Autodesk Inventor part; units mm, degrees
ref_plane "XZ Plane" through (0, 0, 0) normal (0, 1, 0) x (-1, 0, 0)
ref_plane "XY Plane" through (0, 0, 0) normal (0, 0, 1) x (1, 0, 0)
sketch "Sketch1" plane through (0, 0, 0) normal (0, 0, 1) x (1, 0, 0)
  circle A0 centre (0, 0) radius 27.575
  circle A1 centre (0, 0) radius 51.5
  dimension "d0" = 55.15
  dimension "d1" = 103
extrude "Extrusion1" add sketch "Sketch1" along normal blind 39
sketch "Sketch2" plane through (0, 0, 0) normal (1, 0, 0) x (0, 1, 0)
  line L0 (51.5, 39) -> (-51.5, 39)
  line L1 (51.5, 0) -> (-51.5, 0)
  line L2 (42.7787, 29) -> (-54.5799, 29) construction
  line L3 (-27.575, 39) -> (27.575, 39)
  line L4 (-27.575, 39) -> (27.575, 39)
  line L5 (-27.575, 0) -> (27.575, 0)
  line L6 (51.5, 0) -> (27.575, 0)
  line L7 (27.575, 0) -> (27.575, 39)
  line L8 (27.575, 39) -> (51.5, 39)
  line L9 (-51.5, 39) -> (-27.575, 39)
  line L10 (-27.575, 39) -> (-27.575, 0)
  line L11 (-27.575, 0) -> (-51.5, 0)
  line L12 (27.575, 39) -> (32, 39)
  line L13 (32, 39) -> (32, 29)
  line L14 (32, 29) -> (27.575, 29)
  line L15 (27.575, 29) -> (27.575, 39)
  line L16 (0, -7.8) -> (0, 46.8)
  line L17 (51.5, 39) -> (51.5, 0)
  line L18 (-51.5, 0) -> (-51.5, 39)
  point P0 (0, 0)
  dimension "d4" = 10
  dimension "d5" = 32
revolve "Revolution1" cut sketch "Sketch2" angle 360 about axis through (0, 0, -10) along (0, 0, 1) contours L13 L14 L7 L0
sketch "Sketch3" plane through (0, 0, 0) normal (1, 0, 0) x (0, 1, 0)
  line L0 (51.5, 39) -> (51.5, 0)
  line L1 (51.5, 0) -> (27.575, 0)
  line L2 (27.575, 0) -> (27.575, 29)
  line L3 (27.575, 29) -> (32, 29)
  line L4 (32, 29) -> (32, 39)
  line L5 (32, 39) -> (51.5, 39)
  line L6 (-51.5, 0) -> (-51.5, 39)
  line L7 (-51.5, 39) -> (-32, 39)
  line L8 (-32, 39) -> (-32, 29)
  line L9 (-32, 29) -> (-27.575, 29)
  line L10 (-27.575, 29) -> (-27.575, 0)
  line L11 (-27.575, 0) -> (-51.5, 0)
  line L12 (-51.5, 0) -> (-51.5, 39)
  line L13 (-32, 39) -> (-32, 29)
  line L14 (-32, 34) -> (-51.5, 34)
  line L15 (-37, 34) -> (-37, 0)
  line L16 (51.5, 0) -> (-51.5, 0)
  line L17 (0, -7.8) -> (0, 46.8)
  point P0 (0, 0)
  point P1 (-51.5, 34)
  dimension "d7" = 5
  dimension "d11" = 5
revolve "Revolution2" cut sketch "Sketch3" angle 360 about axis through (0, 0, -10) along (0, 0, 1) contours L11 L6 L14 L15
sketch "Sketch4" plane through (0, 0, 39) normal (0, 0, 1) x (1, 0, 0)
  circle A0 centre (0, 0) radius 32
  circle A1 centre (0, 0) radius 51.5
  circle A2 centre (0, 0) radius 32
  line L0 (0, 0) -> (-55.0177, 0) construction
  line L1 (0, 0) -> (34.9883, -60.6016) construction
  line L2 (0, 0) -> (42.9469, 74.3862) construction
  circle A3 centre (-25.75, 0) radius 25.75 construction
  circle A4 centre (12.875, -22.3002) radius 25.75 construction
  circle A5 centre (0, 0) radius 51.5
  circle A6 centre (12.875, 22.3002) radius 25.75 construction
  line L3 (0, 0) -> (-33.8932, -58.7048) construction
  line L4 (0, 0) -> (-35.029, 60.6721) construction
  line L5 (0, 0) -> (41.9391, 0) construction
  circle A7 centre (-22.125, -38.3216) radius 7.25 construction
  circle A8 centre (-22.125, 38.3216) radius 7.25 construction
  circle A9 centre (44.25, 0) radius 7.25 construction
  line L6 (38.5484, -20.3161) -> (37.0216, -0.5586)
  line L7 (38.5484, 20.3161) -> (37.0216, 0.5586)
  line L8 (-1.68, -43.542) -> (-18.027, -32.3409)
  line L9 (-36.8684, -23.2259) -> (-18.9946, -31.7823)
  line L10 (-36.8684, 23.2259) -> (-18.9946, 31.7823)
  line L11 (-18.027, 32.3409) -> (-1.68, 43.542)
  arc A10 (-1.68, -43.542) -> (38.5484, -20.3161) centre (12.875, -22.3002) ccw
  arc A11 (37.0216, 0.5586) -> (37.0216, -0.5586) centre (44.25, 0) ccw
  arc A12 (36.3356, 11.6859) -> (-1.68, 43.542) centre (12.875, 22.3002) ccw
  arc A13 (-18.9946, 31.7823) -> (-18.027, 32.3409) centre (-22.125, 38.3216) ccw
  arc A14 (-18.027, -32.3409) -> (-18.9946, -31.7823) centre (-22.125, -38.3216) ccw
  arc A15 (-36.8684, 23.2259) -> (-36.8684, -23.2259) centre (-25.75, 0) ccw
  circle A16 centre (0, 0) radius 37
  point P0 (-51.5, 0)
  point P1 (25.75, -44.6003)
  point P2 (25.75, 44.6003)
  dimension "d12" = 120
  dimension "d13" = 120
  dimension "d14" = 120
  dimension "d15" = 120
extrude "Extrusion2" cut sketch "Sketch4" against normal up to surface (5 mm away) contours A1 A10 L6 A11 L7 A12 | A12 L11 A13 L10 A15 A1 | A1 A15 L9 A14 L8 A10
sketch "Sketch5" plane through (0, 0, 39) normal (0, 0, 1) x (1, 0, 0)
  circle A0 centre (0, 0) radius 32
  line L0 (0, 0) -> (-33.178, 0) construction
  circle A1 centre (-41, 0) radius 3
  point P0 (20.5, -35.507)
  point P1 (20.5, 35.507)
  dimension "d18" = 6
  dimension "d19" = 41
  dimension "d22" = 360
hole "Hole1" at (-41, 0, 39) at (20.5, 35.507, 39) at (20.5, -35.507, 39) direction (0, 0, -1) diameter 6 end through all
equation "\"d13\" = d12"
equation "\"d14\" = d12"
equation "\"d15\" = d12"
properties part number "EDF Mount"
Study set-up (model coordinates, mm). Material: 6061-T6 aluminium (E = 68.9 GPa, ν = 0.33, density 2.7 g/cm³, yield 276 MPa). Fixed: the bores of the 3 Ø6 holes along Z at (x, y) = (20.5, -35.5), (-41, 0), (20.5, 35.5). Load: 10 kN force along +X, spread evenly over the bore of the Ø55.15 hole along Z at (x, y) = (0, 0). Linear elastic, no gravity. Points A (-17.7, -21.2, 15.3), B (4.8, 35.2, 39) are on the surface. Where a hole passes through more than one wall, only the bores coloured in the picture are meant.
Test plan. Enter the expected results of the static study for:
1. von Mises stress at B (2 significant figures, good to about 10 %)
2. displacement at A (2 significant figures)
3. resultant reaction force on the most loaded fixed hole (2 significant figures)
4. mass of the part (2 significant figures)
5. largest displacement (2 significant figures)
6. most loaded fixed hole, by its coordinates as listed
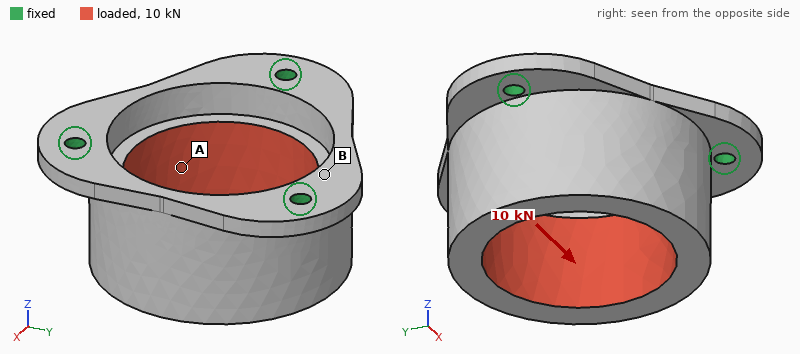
21 MPa
28 µm
4.8 kN
200 g
77 µm
(-41, 0)
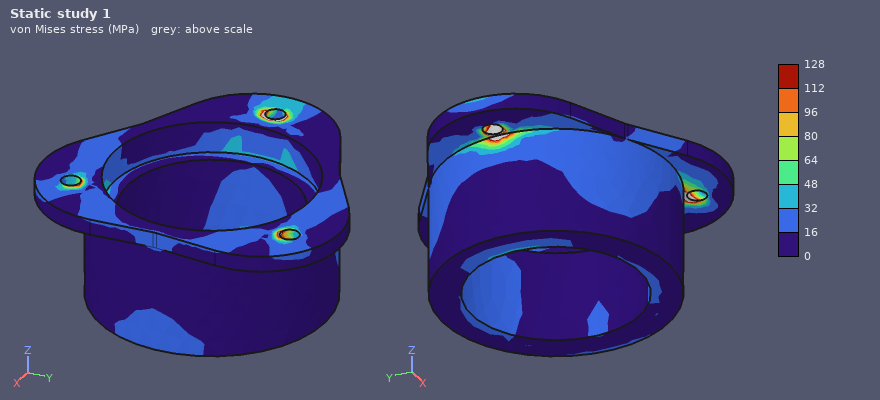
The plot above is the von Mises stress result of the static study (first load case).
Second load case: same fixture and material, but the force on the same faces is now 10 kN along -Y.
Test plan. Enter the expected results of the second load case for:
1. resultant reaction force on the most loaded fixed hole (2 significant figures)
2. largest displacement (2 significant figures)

4.5 kN
68 µm
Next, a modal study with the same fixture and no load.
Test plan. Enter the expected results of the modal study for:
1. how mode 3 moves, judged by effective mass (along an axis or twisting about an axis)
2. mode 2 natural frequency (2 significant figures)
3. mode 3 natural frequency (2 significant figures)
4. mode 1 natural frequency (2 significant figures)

along Z
5100 Hz
8500 Hz
5100 Hz
